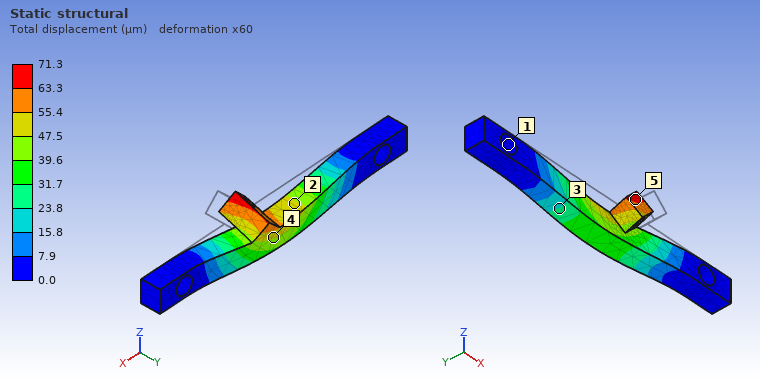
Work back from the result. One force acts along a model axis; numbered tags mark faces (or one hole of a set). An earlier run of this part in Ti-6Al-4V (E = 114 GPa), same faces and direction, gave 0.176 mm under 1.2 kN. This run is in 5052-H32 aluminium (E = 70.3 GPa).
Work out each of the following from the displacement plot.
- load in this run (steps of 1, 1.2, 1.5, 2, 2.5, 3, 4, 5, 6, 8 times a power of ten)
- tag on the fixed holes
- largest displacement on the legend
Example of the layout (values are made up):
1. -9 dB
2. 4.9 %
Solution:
1. 300 N
2. 1
3. 71.3 µm
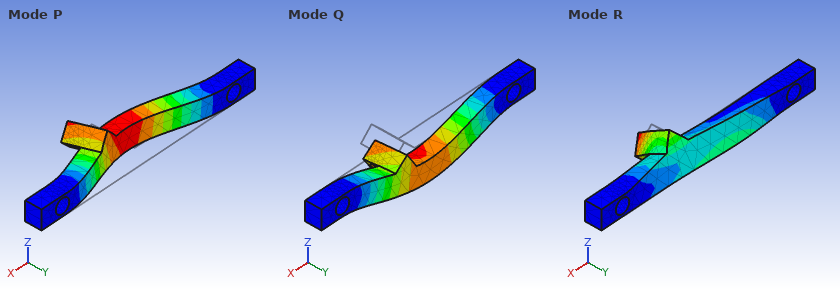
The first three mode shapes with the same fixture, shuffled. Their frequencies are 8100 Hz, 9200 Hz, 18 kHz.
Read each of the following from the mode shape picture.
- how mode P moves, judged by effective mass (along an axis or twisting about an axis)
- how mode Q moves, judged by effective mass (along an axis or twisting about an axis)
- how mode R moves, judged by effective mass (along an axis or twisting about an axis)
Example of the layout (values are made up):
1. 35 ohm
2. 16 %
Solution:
1. along Y
2. along Z
3. twisting about X
